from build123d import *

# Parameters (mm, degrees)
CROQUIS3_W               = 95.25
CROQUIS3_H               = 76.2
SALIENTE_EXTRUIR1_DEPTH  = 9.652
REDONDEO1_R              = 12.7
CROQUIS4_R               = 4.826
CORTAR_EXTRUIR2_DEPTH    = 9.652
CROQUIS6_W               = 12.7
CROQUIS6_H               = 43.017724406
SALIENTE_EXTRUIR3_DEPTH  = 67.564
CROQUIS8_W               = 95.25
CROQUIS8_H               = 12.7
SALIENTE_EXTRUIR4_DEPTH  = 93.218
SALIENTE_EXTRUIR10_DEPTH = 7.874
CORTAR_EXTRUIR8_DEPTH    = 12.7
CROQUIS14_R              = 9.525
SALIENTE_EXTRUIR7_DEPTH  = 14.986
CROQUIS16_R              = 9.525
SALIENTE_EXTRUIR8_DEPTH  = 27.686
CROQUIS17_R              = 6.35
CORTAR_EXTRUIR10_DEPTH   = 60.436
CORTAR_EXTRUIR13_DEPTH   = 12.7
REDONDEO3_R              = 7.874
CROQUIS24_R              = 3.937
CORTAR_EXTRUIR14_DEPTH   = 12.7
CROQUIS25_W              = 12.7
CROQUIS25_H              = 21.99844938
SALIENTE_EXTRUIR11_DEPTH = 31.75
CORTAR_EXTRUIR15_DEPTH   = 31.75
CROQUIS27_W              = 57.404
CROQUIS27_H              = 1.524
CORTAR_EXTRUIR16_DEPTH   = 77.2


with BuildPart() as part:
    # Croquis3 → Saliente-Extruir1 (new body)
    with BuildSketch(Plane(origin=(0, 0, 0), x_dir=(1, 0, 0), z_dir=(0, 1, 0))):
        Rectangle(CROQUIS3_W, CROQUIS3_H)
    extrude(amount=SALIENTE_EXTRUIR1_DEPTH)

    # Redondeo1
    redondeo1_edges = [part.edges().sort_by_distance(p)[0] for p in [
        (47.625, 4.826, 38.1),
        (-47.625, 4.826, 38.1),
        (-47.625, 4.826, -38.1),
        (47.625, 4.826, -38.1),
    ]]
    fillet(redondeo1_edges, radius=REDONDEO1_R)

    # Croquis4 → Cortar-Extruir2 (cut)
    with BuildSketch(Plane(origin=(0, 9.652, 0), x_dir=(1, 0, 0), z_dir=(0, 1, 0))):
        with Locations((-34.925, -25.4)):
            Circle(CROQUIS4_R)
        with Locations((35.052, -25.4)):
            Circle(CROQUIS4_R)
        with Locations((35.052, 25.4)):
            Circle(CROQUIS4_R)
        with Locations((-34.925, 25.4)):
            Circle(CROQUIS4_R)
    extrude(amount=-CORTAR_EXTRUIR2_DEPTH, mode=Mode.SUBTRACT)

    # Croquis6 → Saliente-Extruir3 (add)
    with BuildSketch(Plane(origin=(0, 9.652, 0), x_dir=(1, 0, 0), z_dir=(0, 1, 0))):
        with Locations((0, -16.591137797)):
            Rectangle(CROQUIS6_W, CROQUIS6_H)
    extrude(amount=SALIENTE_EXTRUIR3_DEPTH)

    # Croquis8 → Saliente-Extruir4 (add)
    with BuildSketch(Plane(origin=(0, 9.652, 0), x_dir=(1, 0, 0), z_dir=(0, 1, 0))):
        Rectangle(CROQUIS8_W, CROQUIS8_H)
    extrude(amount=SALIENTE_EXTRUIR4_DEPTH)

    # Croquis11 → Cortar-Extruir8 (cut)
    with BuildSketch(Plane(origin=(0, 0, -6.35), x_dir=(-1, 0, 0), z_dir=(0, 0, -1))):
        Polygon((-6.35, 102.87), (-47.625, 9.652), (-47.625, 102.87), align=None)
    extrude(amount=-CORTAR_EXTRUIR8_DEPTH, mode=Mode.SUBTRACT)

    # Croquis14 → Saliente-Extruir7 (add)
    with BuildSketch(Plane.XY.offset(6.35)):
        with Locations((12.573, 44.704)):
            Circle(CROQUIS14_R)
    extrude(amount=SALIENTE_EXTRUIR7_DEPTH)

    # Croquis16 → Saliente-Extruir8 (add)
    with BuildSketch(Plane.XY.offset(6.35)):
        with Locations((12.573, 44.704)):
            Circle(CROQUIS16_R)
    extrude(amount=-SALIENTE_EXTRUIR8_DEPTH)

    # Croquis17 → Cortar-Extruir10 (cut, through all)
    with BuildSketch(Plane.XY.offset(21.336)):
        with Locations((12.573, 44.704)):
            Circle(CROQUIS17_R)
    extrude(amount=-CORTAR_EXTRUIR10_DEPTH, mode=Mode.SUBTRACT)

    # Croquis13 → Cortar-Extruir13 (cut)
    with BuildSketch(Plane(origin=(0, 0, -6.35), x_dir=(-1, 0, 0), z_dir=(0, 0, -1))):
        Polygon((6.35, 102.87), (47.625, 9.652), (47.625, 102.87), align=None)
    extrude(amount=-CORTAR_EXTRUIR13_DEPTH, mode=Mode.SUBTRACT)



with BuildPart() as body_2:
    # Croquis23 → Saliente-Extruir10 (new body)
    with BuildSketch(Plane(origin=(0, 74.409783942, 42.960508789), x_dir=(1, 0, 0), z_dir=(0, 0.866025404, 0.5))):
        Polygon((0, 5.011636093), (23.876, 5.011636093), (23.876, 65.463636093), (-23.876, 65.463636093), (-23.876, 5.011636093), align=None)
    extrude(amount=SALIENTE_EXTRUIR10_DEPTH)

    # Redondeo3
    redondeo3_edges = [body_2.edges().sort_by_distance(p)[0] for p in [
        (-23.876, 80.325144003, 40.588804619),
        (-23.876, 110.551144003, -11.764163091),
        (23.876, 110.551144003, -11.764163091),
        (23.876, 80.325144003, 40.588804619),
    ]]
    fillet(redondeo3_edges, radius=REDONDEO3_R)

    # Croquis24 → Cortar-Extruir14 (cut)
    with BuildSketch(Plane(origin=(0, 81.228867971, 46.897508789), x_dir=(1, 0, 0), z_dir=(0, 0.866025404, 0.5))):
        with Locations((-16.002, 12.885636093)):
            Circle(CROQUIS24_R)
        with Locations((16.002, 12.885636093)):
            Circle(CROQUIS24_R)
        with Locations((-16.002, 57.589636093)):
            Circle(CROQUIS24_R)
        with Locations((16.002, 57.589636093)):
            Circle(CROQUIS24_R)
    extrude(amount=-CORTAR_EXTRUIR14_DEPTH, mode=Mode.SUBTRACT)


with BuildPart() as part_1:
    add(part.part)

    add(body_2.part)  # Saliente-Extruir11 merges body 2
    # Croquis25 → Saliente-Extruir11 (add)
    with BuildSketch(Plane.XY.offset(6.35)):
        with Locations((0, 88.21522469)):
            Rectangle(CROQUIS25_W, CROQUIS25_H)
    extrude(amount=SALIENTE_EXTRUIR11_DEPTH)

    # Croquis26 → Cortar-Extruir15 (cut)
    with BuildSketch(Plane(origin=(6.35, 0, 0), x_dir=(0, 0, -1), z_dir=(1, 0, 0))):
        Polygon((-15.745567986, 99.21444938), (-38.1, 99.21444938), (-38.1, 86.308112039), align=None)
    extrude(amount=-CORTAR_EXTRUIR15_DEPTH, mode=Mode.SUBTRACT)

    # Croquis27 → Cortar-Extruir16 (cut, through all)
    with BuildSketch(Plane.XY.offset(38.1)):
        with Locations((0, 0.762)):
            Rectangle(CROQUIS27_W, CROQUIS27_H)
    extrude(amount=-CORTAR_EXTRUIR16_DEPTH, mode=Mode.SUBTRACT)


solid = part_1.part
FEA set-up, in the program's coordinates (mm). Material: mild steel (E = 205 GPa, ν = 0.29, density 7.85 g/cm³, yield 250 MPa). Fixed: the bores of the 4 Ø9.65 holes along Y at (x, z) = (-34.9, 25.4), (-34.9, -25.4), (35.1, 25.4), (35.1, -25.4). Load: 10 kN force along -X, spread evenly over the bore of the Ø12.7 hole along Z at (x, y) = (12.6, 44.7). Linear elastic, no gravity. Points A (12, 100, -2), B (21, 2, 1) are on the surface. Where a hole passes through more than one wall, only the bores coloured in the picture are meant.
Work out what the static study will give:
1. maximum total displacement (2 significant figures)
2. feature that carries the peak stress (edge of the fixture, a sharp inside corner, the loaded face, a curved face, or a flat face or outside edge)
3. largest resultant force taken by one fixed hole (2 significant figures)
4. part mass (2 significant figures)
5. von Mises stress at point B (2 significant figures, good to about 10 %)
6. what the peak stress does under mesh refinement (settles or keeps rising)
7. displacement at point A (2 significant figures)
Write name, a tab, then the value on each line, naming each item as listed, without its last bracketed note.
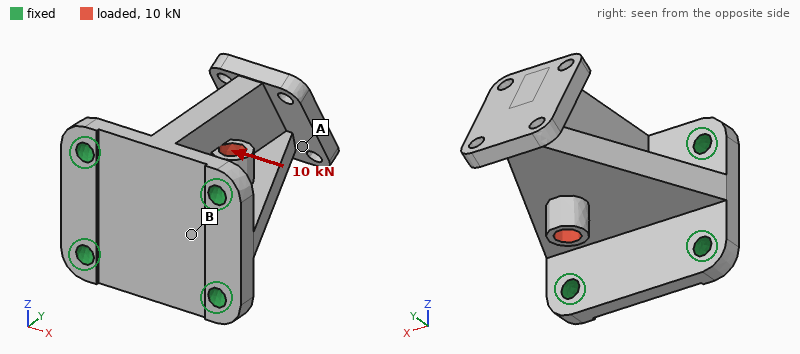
maximum total displacement	32 µm
feature that carries the peak stress	edge of the fixture
largest resultant force taken by one fixed hole	4.2 kN
part mass	1.4 kg
von Mises stress at point B	13 MPa
what the peak stress does under mesh refinement	keeps rising
displacement at point A	28 µm
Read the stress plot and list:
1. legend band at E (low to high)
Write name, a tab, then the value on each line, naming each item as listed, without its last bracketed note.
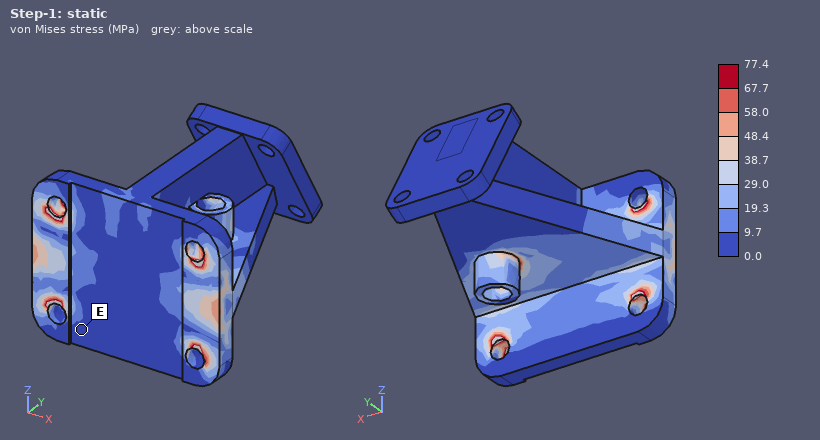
legend band at E	0.0 to 9.7 MPa
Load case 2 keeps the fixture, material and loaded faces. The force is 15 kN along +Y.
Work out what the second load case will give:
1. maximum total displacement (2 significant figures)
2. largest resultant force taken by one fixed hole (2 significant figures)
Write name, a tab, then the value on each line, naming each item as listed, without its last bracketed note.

maximum total displacement	35 µm
largest resultant force taken by one fixed hole	5.4 kN
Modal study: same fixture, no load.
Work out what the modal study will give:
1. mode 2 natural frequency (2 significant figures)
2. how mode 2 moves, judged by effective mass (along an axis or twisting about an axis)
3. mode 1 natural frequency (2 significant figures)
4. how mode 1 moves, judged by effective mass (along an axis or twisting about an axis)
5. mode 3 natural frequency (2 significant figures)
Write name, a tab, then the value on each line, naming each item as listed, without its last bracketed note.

mode 2 natural frequency	2700 Hz
how mode 2 moves, judged by effective mass	along X
mode 1 natural frequency	1500 Hz
how mode 1 moves, judged by effective mass	along Z
mode 3 natural frequency	4200 Hz
